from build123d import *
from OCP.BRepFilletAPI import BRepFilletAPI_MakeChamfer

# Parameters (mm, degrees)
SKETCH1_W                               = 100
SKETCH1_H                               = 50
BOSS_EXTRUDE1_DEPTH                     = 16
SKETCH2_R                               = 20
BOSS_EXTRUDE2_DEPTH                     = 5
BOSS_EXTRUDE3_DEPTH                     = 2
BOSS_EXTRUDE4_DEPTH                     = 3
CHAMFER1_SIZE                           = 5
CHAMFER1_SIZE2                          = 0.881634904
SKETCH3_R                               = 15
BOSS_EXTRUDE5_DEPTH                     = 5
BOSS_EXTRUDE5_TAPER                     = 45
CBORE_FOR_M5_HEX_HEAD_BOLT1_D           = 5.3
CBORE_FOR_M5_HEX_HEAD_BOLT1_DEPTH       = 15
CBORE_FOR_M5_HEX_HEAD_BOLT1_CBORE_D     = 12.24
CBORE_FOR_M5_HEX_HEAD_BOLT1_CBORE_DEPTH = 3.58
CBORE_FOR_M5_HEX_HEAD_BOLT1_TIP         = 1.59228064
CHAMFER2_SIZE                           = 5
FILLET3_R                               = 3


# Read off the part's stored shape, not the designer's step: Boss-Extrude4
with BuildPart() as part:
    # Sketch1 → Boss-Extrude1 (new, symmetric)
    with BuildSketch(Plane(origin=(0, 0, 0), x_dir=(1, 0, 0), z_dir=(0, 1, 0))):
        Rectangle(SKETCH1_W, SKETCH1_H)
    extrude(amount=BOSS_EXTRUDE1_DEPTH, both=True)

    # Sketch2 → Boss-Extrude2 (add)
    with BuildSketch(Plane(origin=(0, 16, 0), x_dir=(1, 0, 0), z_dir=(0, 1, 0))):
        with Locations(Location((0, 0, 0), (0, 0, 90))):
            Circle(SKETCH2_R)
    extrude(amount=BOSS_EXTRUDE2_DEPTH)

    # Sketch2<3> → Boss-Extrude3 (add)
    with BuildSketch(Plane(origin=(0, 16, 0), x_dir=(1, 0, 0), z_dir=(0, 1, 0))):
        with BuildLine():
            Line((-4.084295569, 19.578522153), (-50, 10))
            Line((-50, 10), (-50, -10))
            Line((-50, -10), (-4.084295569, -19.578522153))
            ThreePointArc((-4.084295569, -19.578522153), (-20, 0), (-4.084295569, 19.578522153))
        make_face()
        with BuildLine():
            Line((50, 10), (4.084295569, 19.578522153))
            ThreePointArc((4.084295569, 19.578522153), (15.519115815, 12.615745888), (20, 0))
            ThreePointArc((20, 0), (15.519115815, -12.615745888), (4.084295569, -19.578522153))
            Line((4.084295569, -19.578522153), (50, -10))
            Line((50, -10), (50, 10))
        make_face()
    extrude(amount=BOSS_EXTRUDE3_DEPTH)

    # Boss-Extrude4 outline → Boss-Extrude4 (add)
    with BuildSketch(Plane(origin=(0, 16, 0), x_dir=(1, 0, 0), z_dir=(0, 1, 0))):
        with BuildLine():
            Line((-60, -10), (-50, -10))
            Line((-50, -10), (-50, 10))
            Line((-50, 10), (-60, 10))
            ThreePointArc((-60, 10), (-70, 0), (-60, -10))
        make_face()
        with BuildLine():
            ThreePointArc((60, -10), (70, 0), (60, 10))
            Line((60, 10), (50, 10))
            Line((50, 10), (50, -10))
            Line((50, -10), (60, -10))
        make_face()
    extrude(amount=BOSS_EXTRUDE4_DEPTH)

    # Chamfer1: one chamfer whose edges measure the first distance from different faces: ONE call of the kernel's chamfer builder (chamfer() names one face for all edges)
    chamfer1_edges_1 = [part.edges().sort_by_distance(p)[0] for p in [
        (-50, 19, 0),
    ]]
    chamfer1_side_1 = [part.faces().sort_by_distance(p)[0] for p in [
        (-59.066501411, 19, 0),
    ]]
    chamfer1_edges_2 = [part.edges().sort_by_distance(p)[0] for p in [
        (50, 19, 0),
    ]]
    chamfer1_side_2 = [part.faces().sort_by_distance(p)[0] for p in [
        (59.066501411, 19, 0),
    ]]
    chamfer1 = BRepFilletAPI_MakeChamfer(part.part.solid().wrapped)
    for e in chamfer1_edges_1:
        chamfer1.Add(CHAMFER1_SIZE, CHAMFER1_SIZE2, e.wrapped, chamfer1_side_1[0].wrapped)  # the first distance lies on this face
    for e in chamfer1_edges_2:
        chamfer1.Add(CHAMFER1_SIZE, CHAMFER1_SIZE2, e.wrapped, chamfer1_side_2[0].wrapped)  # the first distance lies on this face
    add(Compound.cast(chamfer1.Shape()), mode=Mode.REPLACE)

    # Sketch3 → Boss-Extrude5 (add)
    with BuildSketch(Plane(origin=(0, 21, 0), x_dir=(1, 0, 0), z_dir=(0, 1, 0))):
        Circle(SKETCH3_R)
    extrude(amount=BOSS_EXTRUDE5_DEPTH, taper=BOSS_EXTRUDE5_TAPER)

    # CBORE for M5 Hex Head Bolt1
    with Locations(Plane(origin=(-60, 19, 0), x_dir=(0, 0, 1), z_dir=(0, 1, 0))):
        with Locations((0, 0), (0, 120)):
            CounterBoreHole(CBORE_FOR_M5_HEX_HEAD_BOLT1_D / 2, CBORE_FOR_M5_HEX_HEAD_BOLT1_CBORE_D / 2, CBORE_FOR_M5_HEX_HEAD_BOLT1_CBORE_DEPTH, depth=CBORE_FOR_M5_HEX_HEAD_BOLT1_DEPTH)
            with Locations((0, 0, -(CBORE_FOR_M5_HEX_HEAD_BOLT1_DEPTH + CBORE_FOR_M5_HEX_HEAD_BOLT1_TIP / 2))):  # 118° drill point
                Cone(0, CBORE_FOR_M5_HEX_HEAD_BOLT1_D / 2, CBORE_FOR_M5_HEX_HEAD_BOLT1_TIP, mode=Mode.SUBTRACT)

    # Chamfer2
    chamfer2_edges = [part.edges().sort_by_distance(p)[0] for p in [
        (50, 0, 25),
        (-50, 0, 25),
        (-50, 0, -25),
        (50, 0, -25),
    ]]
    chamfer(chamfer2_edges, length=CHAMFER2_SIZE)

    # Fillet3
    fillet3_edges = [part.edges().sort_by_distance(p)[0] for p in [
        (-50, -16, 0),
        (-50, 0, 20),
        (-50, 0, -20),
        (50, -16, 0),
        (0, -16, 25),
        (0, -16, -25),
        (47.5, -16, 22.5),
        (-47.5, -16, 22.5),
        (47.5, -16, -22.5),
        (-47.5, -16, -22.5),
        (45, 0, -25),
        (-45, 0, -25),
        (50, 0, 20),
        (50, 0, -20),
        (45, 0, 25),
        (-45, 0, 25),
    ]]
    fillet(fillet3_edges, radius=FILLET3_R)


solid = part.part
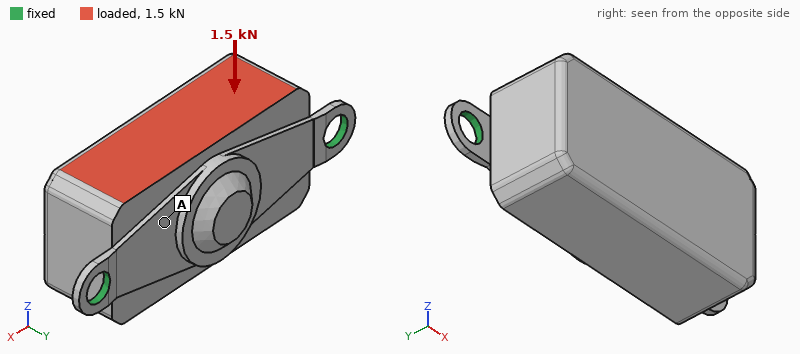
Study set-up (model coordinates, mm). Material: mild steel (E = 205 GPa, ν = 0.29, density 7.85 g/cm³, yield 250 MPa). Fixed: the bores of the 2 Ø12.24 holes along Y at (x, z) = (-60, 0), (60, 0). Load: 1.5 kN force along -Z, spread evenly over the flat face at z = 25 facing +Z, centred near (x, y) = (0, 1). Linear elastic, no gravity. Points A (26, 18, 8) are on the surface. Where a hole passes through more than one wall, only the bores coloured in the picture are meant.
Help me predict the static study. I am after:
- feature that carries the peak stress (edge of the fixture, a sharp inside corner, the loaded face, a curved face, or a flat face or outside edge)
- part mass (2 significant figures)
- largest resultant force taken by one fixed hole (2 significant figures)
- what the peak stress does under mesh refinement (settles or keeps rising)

edge of the fixture
1.3 kg
750 N
keeps rising
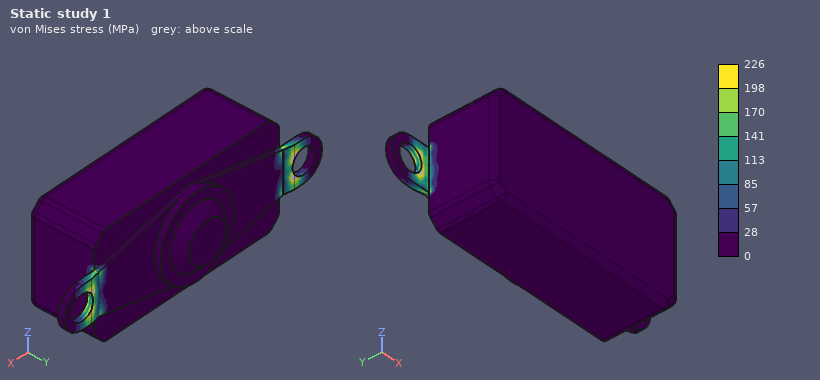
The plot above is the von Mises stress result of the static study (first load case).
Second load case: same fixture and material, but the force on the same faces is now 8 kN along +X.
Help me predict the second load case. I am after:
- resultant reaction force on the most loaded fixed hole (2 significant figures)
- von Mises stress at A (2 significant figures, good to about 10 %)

4.6 kN
11 MPa
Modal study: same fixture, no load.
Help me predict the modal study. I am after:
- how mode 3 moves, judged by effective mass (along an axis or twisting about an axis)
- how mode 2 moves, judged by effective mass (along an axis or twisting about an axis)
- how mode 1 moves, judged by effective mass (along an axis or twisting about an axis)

along X
along Y
along Z
